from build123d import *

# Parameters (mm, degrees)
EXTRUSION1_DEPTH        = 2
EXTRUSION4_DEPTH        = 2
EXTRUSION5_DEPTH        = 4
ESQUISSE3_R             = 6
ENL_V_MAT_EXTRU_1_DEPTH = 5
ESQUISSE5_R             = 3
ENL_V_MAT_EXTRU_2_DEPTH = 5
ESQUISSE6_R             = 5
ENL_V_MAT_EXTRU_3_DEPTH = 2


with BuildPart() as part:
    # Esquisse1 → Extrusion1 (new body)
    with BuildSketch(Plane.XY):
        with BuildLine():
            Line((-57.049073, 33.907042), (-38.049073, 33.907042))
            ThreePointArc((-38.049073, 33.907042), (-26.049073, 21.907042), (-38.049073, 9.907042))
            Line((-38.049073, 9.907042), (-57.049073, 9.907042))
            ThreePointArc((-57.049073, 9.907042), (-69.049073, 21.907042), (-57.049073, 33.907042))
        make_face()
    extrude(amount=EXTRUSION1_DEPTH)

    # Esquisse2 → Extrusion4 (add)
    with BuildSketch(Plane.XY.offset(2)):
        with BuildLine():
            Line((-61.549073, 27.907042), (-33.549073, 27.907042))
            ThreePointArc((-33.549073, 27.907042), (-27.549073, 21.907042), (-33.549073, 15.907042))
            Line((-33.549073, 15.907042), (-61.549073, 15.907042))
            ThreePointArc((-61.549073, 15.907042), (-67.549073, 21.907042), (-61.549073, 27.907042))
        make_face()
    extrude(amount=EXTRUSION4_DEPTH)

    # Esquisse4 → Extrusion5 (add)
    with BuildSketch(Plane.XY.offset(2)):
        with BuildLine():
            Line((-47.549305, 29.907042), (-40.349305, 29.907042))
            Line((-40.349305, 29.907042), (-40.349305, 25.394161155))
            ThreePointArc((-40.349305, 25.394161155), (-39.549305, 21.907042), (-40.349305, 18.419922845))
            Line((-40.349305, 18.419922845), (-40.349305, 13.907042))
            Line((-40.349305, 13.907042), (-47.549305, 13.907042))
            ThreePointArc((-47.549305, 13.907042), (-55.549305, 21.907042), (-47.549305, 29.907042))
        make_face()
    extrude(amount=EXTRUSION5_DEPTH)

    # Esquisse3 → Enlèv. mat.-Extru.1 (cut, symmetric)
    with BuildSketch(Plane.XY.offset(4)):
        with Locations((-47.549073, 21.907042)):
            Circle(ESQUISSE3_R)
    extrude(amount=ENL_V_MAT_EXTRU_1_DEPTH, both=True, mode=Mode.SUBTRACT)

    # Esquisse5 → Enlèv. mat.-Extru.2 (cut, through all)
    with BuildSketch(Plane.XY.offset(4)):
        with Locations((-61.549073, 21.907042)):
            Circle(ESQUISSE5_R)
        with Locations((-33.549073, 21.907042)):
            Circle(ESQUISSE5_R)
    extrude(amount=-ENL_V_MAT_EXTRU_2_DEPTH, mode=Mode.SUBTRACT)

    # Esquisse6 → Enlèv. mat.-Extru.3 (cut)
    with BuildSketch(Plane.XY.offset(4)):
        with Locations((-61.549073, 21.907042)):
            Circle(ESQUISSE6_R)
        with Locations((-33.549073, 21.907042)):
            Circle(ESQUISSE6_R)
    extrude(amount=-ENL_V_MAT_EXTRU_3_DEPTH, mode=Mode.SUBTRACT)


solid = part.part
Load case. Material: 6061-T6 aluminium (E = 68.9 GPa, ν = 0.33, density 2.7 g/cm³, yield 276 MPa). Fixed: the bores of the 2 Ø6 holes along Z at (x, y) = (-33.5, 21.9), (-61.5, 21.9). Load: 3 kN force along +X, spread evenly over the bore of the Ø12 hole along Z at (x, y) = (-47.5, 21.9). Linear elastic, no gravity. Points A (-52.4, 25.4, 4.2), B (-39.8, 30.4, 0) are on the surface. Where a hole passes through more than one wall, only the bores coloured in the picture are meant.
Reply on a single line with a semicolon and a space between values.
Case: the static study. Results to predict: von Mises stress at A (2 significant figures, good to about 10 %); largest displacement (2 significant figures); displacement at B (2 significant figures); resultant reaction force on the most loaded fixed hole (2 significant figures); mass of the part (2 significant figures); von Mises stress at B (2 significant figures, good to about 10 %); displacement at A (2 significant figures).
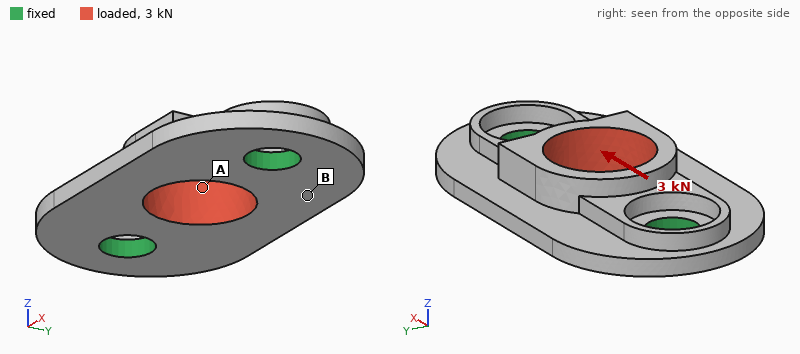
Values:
34 MPa; 10 µm; 4.6 µm; 1.5 kN; 5.8 g; 15 MPa; 7.3 µm
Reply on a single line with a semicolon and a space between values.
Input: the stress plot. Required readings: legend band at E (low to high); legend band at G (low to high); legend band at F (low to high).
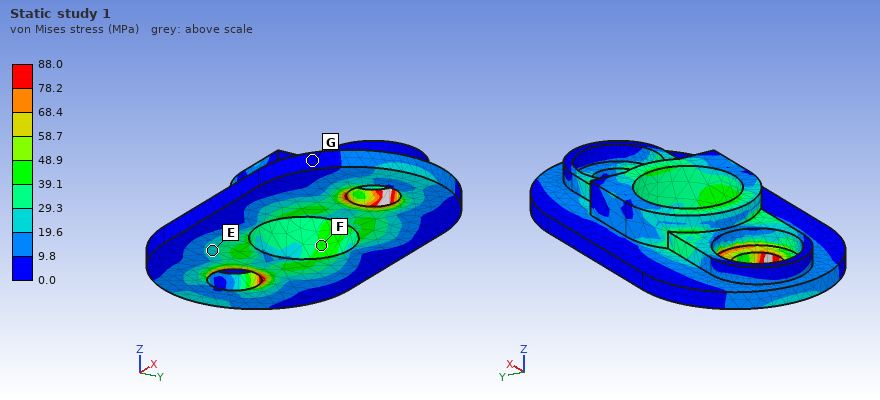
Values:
19.6 to 29.3 MPa; 0.0 to 9.8 MPa; 39.1 to 48.9 MPa
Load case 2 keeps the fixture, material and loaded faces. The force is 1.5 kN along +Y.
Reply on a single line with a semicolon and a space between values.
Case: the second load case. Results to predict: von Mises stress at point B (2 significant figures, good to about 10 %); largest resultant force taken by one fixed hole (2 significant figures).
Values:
21 MPa; 750 N
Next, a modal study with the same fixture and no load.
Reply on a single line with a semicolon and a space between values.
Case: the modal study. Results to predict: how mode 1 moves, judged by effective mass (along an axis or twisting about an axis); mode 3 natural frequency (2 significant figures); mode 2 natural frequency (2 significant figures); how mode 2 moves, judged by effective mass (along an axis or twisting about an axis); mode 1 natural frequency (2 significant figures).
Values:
twisting about X; 26 kHz; 18 kHz; along Z; 13 kHz
